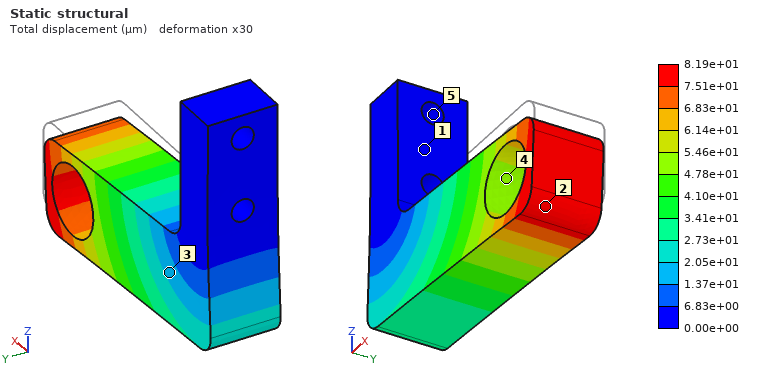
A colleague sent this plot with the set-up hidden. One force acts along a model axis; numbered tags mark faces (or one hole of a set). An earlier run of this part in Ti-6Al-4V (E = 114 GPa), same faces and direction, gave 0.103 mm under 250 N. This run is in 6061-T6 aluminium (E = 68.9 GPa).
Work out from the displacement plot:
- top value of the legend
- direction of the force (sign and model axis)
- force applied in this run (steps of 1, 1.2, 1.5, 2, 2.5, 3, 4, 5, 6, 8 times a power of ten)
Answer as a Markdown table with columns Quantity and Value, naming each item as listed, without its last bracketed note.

| Quantity | Value |
|---|---|
| top value of the legend | 8.19e+01 µm |
| direction of the force | -Z |
| force applied in this run | 120 N |
